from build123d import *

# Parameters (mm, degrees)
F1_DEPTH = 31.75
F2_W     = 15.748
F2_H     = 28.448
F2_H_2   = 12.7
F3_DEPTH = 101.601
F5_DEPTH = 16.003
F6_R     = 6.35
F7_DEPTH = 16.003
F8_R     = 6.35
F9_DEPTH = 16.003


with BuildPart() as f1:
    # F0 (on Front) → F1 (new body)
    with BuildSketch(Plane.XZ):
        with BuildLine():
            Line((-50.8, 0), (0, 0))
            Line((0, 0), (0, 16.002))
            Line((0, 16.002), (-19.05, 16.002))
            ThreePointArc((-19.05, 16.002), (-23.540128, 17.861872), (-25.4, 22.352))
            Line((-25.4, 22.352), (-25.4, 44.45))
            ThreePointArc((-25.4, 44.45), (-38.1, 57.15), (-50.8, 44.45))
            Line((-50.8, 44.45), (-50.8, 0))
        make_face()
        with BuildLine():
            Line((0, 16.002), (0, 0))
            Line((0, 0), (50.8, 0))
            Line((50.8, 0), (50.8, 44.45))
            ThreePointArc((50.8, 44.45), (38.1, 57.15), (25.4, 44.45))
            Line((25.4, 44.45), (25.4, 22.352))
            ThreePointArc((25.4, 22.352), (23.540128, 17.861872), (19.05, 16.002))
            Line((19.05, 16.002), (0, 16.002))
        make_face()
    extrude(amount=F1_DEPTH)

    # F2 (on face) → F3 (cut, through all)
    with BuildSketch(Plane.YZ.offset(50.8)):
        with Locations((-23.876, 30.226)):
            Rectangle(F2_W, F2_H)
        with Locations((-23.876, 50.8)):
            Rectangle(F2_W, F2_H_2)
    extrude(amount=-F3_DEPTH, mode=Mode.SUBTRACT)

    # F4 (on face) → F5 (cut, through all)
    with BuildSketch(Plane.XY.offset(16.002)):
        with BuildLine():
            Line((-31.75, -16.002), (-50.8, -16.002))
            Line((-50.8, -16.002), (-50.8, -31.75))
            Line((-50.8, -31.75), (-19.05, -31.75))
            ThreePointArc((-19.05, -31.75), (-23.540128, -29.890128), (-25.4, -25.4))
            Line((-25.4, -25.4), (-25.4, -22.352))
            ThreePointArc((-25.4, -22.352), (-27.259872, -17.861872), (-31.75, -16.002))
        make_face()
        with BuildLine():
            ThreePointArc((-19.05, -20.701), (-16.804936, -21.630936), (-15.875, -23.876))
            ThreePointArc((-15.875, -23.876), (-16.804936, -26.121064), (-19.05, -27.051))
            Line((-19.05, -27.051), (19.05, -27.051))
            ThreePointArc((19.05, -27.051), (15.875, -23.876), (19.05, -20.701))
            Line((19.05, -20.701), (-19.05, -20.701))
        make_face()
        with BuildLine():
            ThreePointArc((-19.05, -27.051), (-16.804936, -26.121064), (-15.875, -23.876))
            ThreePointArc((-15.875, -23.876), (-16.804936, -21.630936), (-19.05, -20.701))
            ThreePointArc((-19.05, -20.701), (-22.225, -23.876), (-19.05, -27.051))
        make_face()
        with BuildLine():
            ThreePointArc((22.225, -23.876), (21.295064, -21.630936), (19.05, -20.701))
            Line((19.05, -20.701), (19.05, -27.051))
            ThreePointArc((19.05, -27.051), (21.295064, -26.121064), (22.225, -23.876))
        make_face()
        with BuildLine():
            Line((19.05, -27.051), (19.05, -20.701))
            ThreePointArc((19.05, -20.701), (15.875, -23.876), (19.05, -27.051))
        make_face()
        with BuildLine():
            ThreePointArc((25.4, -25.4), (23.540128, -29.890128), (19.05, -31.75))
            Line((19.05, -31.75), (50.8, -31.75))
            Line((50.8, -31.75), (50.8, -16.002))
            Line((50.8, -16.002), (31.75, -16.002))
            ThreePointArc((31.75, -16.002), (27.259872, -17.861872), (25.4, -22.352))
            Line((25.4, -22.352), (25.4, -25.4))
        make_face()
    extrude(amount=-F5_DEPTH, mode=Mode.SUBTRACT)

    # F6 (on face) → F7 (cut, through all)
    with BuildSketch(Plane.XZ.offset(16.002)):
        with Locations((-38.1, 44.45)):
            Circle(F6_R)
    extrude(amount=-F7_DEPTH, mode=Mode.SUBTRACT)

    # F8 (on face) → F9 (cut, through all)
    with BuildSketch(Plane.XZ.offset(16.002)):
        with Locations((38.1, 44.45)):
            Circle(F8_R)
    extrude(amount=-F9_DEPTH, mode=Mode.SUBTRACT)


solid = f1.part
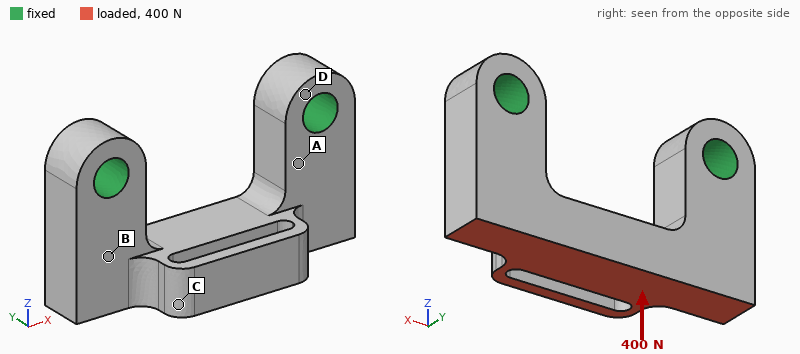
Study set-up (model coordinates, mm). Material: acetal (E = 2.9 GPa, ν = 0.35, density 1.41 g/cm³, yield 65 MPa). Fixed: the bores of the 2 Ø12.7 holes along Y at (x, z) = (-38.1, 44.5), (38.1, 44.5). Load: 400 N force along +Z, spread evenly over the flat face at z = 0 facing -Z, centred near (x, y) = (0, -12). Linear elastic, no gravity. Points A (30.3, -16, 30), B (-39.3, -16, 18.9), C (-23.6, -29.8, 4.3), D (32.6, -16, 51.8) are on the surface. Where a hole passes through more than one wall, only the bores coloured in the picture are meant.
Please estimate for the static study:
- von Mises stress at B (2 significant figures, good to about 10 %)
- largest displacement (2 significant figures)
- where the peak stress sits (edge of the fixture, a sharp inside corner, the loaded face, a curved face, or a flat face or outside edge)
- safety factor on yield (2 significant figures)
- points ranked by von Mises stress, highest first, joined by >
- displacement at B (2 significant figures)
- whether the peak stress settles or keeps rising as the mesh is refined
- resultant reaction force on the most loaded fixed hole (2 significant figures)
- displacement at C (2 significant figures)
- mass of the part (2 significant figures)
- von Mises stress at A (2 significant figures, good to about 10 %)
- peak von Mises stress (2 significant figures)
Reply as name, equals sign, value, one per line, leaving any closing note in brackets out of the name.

von Mises stress at B = 0.83 MPa
largest displacement = 72 µm
where the peak stress sits = a curved face
safety factor on yield = 16
points ranked by von Mises stress, highest first, joined by > = A > B > C > D
displacement at B = 12 µm
whether the peak stress settles or keeps rising as the mesh is refined = settles
resultant reaction force on the most loaded fixed hole = 210 N
displacement at C = 53 µm
mass of the part = 87 g
von Mises stress at A = 1.6 MPa
peak von Mises stress = 4.0 MPa
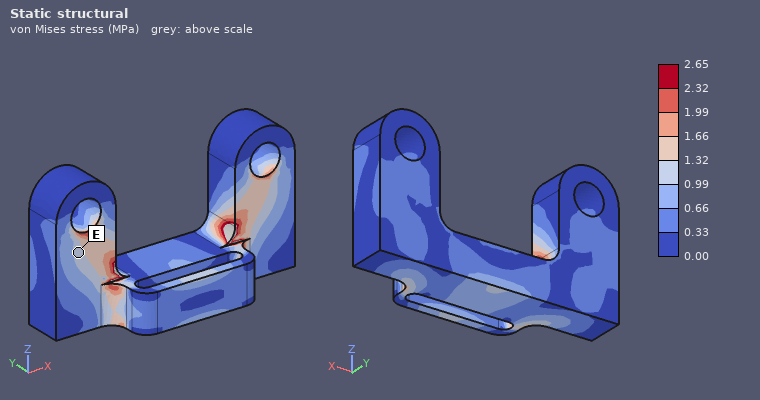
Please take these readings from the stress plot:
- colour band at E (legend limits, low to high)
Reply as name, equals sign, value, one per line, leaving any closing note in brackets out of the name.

colour band at E = 0.99 to 1.32 MPa
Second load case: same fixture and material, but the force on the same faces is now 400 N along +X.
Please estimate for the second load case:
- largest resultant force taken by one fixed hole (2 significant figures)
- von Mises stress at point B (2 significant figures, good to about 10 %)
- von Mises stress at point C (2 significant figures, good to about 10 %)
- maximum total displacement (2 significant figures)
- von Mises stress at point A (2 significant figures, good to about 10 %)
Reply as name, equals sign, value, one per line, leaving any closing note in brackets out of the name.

largest resultant force taken by one fixed hole = 230 N
von Mises stress at point B = 0.95 MPa
von Mises stress at point C = 0.63 MPa
maximum total displacement = 65 µm
von Mises stress at point A = 1.0 MPa
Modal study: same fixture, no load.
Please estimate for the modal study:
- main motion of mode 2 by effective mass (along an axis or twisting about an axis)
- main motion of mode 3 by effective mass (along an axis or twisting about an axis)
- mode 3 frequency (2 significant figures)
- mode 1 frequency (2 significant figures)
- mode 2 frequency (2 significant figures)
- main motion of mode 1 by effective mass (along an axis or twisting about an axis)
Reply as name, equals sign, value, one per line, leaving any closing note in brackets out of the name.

main motion of mode 2 by effective mass = along X
main motion of mode 3 by effective mass = along X
mode 3 frequency = 2200 Hz
mode 1 frequency = 1200 Hz
mode 2 frequency = 2000 Hz
main motion of mode 1 by effective mass = along Y
